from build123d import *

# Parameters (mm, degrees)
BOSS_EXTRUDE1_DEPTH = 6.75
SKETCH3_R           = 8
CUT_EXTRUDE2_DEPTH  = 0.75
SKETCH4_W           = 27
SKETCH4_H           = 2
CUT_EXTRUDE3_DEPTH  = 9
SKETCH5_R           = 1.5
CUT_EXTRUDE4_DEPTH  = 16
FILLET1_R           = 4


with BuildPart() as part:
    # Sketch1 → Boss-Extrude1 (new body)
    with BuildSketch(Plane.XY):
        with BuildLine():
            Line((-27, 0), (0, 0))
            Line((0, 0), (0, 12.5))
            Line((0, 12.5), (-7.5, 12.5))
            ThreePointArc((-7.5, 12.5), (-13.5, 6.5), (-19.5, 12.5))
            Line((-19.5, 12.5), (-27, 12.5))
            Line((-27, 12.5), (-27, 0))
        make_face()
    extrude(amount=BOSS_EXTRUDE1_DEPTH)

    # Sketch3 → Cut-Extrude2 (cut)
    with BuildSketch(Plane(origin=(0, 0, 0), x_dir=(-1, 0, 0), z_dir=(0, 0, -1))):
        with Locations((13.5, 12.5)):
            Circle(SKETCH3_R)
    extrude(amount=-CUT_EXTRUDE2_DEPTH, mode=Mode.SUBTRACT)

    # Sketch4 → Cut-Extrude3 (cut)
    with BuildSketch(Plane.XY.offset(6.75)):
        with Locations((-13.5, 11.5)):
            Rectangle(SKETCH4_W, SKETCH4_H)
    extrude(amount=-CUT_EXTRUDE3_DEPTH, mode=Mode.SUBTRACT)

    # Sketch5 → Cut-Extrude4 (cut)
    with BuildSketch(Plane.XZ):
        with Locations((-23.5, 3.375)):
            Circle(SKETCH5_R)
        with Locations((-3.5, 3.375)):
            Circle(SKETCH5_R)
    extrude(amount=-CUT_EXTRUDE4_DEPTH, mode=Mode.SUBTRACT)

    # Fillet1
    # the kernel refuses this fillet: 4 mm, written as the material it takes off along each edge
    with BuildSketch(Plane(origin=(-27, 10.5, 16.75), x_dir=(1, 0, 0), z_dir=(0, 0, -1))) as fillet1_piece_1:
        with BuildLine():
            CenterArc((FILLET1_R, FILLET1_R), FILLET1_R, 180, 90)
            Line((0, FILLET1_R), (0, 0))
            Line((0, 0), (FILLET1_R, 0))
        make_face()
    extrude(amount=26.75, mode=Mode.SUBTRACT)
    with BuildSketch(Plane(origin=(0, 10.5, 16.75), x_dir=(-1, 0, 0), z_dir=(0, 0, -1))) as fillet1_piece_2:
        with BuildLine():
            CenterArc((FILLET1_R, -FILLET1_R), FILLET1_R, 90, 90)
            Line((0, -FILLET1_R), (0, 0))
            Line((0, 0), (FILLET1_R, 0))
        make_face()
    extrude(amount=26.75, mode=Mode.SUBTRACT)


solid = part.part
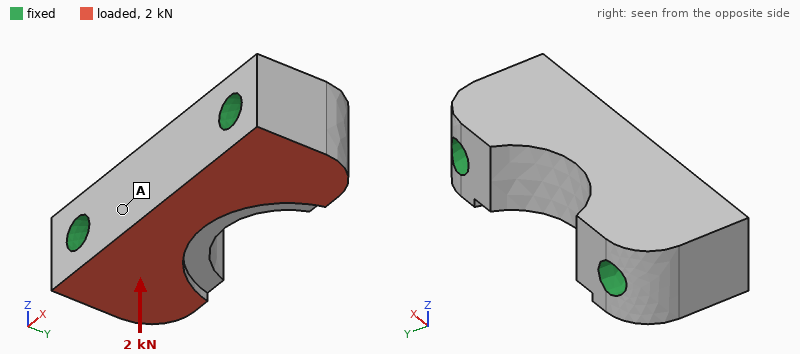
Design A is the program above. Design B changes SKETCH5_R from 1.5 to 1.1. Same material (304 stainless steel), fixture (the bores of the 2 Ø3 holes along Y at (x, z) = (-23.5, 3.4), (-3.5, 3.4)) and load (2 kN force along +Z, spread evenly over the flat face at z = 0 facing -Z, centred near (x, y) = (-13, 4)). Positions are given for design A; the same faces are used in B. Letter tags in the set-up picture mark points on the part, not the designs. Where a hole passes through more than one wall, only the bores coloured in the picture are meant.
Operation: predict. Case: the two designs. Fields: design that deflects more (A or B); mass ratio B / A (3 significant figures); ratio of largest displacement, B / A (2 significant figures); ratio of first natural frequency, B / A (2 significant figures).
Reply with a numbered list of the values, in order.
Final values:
1. B
2. 1.05
3. 1.2
4. 0.87
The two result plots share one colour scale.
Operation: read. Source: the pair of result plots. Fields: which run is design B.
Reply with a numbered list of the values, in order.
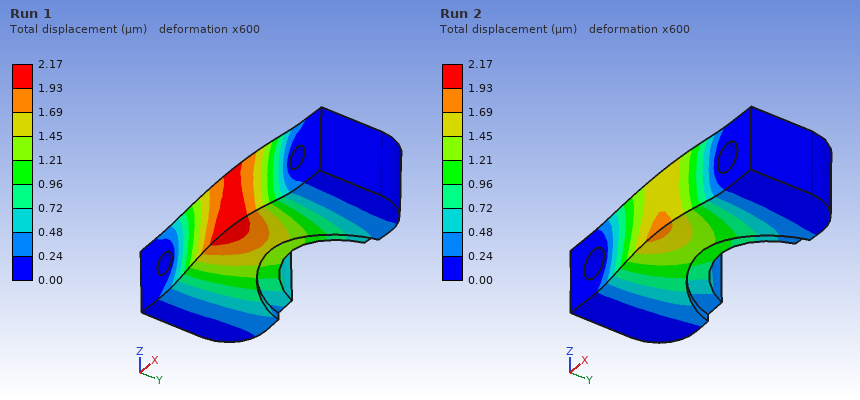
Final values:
1. Run 1
